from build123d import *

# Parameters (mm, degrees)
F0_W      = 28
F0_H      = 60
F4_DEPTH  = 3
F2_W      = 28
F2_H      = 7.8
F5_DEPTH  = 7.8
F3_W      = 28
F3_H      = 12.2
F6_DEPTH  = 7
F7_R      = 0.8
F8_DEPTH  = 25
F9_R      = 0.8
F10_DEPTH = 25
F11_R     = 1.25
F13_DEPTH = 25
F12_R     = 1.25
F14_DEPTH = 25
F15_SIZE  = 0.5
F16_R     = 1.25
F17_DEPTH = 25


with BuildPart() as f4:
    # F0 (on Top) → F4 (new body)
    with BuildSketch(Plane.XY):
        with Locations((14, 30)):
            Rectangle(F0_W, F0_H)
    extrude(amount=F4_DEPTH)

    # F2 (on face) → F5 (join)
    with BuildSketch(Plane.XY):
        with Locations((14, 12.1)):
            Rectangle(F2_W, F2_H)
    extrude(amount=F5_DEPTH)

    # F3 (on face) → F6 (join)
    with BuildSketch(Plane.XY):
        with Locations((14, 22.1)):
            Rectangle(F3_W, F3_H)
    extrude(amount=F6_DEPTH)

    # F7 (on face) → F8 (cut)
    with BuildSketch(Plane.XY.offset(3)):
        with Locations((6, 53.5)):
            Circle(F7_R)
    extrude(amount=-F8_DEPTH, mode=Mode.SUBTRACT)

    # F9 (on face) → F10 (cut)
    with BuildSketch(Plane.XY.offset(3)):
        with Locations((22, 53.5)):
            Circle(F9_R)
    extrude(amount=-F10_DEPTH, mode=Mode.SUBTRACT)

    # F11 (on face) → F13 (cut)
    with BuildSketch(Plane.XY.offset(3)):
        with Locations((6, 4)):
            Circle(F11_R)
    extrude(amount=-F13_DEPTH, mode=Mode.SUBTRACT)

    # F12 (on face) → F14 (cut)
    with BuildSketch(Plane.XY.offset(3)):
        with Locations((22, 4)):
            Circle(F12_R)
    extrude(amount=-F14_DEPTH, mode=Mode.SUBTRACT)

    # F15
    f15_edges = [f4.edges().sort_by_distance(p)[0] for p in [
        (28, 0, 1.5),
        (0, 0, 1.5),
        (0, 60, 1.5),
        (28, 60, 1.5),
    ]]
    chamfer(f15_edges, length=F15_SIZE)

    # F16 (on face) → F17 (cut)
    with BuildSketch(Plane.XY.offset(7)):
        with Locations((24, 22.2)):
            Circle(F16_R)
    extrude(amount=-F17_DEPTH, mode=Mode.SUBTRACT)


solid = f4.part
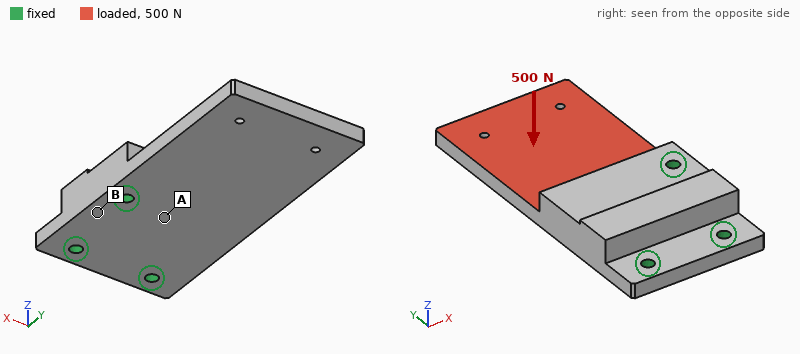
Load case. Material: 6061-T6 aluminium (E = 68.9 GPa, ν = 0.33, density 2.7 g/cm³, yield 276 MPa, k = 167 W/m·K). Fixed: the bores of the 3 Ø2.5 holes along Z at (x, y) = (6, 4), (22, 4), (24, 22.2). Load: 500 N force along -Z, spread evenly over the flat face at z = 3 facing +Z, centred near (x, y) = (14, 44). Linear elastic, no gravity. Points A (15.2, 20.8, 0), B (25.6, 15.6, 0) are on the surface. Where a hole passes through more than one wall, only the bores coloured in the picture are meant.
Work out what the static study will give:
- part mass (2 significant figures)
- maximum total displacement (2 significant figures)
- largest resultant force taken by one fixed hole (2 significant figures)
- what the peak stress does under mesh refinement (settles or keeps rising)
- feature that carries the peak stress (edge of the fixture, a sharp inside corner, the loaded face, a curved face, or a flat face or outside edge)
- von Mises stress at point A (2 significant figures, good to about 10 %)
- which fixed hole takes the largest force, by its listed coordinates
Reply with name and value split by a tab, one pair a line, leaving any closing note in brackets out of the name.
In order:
part mass	20 g
maximum total displacement	0.63 mm
largest resultant force taken by one fixed hole	800 N
what the peak stress does under mesh refinement	keeps rising
feature that carries the peak stress	edge of the fixture
von Mises stress at point A	37 MPa
which fixed hole takes the largest force, by its listed coordinates	(24, 22.2)
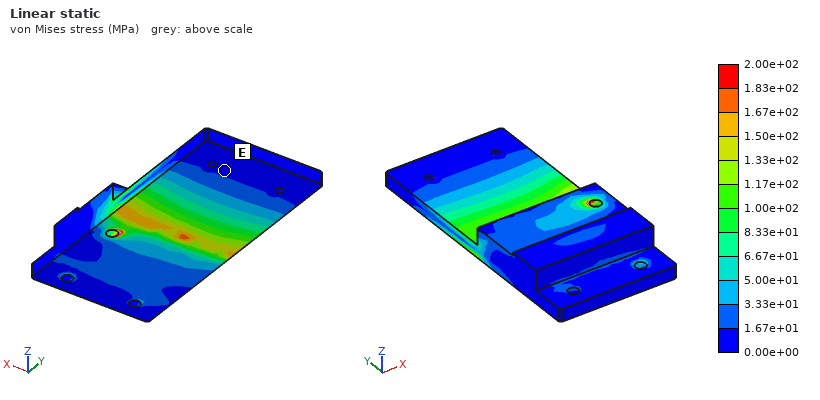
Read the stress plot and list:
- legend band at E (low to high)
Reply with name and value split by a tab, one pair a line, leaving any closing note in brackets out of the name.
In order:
legend band at E	0.00e+00 to 1.67e+01 MPa
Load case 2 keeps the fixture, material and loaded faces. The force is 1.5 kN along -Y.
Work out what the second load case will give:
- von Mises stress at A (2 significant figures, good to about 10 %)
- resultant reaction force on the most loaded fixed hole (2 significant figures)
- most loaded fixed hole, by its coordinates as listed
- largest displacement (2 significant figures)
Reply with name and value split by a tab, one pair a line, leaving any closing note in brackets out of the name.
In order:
von Mises stress at A	9.3 MPa
resultant reaction force on the most loaded fixed hole	810 N
most loaded fixed hole, by its coordinates as listed	(24, 22.2)
largest displacement	0.19 mm
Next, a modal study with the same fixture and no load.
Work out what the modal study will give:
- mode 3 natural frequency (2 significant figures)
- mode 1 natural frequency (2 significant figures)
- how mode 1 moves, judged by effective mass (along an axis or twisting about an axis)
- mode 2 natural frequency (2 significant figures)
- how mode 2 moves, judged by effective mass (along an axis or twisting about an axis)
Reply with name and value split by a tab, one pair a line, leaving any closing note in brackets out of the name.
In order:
mode 3 natural frequency	9300 Hz
mode 1 natural frequency	2100 Hz
how mode 1 moves, judged by effective mass	along Z
mode 2 natural frequency	5500 Hz
how mode 2 moves, judged by effective mass	twisting about Y
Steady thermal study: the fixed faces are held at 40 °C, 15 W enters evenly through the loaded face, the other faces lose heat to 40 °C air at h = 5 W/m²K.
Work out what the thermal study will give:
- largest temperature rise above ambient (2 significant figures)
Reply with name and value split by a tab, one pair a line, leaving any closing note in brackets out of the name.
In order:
largest temperature rise above ambient	24 K
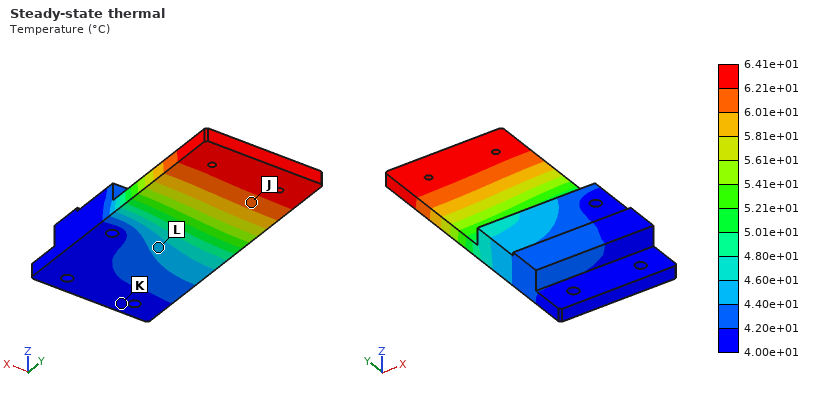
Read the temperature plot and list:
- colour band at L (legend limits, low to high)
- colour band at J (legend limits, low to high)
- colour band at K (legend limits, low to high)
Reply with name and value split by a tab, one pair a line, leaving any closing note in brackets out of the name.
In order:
colour band at L	4.40e+01 to 4.60e+01 °C
colour band at J	6.01e+01 to 6.21e+01 °C
colour band at K	4.00e+01 to 4.20e+01 °C
